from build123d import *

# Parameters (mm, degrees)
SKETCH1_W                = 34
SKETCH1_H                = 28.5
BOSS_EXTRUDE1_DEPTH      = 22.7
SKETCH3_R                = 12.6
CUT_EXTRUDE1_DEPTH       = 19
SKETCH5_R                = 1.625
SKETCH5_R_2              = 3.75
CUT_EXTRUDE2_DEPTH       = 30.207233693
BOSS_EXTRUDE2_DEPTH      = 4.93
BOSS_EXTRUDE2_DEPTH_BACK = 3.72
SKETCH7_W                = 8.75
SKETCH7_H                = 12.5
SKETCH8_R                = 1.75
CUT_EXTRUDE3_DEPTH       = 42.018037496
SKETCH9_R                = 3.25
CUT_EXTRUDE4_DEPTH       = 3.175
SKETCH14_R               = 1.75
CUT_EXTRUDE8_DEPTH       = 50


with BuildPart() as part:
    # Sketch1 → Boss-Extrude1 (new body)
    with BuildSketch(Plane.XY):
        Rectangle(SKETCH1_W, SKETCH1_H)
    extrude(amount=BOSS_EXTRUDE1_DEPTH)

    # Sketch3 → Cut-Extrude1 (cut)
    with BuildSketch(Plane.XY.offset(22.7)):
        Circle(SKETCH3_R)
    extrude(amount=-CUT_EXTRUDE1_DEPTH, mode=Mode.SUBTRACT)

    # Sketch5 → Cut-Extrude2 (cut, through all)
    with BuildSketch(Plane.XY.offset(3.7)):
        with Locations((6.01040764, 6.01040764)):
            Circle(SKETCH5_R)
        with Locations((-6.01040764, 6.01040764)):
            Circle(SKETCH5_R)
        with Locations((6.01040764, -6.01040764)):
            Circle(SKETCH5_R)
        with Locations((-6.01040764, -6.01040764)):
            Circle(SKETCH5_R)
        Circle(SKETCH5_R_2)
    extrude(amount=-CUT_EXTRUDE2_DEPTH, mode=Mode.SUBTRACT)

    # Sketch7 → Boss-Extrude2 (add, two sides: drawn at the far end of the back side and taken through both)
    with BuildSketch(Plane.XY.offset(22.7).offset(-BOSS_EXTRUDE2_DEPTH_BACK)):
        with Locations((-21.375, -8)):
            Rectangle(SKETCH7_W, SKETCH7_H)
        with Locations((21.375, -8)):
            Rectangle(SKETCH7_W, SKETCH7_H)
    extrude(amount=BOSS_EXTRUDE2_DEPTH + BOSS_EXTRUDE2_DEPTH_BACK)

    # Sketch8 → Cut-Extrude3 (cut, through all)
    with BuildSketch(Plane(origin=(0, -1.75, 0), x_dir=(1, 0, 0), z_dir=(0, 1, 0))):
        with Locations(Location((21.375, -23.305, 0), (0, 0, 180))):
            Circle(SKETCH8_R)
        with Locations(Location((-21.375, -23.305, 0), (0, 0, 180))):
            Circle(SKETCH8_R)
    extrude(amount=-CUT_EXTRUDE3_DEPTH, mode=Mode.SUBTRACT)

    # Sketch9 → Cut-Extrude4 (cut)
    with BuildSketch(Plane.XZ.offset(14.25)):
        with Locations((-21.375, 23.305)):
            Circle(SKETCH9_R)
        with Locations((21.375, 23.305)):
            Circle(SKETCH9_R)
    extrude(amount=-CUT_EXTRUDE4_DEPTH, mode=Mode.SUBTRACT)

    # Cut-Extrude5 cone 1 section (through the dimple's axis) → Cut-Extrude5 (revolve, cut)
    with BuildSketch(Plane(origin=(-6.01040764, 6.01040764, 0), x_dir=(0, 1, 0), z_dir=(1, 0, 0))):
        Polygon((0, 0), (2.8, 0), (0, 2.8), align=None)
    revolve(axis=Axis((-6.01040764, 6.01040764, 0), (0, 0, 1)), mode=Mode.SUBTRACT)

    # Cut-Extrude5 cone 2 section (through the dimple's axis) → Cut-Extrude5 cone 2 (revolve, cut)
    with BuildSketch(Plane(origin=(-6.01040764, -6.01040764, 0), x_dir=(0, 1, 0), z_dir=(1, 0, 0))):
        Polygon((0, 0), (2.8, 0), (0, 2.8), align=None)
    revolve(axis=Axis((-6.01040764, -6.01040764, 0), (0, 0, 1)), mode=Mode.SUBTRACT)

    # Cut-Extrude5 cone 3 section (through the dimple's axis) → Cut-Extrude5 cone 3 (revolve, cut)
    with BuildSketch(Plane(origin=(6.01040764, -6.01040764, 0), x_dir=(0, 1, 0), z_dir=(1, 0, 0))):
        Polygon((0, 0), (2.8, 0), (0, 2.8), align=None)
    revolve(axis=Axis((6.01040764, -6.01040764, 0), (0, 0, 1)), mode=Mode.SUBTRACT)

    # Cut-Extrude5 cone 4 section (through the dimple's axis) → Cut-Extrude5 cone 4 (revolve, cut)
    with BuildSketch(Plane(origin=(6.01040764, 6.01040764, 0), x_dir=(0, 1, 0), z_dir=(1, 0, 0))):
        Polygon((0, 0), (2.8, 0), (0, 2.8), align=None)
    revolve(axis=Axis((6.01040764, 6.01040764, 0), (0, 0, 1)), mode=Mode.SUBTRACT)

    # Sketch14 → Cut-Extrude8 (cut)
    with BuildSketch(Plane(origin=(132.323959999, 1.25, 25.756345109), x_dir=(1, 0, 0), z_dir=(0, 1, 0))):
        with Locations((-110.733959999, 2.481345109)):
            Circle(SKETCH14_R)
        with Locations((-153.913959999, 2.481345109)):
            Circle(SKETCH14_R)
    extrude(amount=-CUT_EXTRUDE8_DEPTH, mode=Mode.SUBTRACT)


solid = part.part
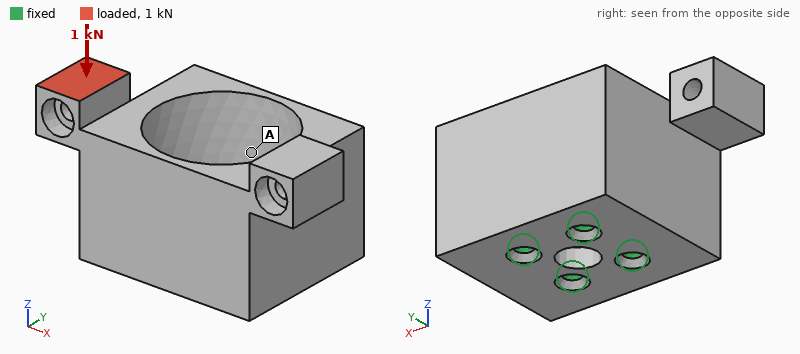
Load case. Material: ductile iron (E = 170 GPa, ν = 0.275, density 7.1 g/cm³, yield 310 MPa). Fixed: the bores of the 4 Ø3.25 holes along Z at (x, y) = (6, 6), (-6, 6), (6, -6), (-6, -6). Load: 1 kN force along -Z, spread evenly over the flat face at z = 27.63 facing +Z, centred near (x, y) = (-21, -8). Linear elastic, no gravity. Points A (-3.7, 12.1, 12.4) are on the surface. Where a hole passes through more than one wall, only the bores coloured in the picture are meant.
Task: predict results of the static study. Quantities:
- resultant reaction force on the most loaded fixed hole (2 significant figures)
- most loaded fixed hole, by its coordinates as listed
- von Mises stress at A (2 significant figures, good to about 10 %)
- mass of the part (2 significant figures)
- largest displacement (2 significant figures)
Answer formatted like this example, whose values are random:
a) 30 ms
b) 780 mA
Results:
a) 1.3 kN
b) (-6, -6)
c) 20 MPa
d) 97 g
e) 59 µm
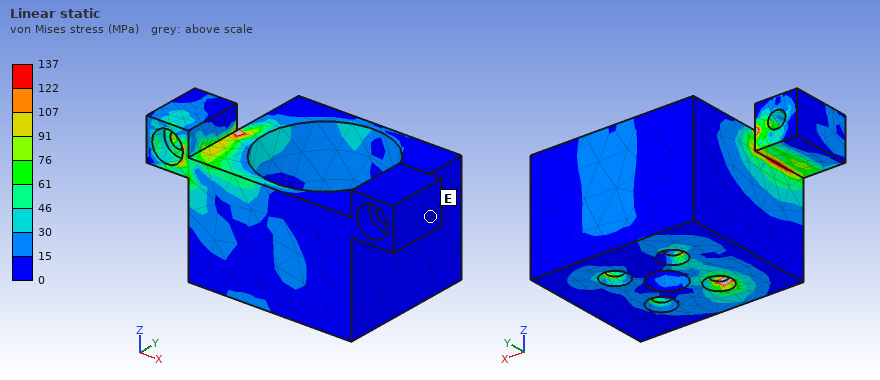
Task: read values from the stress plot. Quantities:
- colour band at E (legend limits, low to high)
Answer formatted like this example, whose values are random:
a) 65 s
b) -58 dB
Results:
a) 0 to 15 MPa
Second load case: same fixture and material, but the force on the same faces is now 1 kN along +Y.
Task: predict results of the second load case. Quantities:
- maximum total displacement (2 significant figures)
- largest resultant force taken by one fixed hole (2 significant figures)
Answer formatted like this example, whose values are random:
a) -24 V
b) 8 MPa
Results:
a) 42 µm
b) 1.4 kN
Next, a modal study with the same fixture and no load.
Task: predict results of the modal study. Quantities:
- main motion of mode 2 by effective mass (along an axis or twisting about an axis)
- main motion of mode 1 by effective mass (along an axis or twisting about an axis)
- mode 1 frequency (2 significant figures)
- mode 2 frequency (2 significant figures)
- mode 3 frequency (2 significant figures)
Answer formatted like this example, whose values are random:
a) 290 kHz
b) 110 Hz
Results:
a) along Y
b) along X
c) 5800 Hz
d) 7000 Hz
e) 9900 Hz
